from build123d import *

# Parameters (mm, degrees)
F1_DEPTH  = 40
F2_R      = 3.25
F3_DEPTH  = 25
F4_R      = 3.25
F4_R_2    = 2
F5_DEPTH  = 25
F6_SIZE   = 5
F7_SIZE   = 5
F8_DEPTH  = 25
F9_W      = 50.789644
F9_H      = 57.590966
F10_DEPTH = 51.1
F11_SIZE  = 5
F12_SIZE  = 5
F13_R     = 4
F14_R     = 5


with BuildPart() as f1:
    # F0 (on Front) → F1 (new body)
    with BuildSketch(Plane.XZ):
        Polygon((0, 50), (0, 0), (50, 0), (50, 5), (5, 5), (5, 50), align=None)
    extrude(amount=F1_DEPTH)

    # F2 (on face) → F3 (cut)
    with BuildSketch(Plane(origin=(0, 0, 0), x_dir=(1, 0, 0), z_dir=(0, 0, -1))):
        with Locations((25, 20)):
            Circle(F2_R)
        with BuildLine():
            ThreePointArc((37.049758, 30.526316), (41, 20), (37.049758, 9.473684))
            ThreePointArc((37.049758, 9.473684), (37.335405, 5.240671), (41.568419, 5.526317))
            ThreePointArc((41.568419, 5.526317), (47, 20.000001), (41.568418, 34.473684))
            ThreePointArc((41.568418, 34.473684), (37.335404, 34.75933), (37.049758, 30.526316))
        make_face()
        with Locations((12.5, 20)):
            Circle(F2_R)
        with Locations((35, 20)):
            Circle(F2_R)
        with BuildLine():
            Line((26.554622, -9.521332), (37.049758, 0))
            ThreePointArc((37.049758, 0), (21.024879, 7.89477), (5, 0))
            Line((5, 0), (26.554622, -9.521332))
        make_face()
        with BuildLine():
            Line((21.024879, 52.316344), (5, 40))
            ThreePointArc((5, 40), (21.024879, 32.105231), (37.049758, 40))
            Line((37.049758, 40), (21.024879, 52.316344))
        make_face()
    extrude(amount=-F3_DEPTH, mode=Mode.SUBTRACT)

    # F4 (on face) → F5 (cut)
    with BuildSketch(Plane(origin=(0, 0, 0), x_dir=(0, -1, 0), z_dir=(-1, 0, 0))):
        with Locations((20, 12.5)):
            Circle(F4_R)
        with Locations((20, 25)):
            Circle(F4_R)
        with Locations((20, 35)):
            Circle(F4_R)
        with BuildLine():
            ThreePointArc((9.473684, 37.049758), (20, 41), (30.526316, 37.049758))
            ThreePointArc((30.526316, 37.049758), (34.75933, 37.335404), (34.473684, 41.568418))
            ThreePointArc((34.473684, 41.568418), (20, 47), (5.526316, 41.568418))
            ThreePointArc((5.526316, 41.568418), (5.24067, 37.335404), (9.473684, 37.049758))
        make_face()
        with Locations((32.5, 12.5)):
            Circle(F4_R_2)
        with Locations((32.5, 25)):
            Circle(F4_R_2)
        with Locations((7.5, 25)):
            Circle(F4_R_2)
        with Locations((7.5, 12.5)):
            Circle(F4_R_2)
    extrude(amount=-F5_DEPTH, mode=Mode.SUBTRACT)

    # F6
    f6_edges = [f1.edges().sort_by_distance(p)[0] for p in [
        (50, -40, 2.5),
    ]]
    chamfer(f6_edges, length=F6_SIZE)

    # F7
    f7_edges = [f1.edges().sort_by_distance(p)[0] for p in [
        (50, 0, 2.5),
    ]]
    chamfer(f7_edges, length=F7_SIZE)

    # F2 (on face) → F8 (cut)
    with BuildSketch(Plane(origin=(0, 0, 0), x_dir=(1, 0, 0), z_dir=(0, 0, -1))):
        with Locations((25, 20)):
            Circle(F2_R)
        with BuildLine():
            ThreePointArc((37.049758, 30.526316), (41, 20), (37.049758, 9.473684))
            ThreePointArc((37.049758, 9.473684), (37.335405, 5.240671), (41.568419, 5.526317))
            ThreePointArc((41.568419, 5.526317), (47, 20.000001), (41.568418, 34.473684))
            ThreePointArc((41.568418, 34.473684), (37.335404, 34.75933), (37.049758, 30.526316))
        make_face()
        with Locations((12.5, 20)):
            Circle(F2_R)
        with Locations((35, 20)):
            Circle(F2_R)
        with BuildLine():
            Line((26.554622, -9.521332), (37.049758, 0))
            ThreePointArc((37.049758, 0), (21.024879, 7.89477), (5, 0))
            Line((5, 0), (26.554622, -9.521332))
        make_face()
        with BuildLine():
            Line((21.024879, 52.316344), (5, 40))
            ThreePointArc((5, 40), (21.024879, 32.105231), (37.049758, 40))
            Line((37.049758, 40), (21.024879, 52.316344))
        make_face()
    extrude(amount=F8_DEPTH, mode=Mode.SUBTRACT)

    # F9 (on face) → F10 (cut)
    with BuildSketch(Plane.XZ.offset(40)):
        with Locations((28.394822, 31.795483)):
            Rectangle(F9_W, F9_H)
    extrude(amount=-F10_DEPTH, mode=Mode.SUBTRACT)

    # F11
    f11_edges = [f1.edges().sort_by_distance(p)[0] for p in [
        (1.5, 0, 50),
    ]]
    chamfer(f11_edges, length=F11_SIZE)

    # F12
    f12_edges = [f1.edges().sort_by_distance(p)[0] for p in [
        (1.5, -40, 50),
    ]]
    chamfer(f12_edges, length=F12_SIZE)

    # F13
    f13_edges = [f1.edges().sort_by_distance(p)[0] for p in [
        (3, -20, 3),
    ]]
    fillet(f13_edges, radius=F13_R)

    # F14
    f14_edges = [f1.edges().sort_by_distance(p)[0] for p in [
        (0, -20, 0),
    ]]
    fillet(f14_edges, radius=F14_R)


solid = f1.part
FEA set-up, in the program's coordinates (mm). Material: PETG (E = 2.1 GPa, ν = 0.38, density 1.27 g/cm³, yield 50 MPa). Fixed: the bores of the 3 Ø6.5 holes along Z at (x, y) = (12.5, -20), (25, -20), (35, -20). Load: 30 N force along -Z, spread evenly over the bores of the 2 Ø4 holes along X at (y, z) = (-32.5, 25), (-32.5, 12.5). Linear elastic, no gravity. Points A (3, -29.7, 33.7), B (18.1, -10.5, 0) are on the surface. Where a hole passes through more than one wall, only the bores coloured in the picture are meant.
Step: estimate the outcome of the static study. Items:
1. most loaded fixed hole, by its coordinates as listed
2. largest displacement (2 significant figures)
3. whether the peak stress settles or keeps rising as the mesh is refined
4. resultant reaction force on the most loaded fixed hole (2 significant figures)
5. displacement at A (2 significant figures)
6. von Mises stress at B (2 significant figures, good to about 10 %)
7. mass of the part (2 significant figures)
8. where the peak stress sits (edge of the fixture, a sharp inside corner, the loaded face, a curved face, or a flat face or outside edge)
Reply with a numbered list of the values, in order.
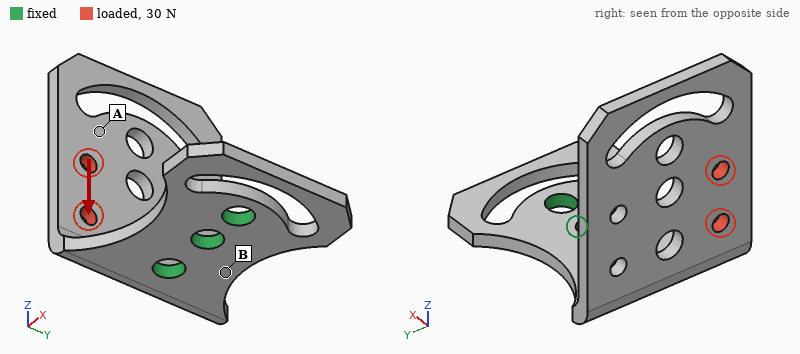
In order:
1. (12.5, -20)
2. 0.77 mm
3. keeps rising
4. 35 N
5. 0.52 mm
6. 2.0 MPa
7. 11 g
8. edge of the fixture
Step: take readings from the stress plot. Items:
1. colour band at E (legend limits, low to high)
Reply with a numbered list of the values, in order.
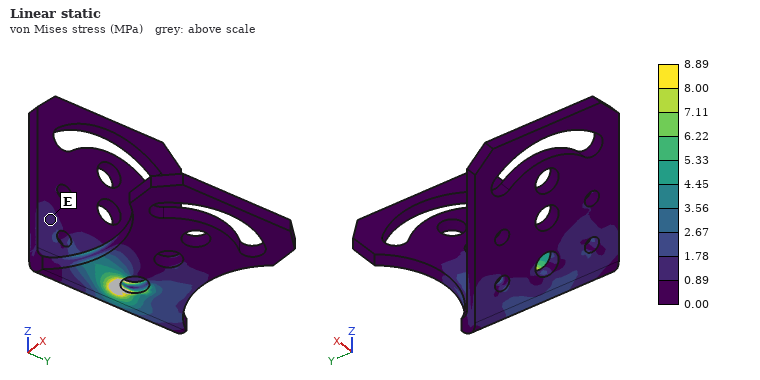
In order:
1. 0.89 to 1.78 MPa
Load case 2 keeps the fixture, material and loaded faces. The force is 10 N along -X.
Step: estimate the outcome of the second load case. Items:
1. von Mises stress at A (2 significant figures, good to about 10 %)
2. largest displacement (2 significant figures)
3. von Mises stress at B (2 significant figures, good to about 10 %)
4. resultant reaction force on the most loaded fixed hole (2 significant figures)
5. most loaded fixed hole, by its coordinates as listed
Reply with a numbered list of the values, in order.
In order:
1. 0.33 MPa
2. 0.83 mm
3. 0.51 MPa
4. 9.3 N
5. (12.5, -20)
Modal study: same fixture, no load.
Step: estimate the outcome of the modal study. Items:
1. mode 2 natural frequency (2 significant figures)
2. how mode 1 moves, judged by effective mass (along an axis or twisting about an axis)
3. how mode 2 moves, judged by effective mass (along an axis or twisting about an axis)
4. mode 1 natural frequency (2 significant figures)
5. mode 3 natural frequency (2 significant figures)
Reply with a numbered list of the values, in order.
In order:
1. 410 Hz
2. along X
3. along Y
4. 240 Hz
5. 710 Hz
